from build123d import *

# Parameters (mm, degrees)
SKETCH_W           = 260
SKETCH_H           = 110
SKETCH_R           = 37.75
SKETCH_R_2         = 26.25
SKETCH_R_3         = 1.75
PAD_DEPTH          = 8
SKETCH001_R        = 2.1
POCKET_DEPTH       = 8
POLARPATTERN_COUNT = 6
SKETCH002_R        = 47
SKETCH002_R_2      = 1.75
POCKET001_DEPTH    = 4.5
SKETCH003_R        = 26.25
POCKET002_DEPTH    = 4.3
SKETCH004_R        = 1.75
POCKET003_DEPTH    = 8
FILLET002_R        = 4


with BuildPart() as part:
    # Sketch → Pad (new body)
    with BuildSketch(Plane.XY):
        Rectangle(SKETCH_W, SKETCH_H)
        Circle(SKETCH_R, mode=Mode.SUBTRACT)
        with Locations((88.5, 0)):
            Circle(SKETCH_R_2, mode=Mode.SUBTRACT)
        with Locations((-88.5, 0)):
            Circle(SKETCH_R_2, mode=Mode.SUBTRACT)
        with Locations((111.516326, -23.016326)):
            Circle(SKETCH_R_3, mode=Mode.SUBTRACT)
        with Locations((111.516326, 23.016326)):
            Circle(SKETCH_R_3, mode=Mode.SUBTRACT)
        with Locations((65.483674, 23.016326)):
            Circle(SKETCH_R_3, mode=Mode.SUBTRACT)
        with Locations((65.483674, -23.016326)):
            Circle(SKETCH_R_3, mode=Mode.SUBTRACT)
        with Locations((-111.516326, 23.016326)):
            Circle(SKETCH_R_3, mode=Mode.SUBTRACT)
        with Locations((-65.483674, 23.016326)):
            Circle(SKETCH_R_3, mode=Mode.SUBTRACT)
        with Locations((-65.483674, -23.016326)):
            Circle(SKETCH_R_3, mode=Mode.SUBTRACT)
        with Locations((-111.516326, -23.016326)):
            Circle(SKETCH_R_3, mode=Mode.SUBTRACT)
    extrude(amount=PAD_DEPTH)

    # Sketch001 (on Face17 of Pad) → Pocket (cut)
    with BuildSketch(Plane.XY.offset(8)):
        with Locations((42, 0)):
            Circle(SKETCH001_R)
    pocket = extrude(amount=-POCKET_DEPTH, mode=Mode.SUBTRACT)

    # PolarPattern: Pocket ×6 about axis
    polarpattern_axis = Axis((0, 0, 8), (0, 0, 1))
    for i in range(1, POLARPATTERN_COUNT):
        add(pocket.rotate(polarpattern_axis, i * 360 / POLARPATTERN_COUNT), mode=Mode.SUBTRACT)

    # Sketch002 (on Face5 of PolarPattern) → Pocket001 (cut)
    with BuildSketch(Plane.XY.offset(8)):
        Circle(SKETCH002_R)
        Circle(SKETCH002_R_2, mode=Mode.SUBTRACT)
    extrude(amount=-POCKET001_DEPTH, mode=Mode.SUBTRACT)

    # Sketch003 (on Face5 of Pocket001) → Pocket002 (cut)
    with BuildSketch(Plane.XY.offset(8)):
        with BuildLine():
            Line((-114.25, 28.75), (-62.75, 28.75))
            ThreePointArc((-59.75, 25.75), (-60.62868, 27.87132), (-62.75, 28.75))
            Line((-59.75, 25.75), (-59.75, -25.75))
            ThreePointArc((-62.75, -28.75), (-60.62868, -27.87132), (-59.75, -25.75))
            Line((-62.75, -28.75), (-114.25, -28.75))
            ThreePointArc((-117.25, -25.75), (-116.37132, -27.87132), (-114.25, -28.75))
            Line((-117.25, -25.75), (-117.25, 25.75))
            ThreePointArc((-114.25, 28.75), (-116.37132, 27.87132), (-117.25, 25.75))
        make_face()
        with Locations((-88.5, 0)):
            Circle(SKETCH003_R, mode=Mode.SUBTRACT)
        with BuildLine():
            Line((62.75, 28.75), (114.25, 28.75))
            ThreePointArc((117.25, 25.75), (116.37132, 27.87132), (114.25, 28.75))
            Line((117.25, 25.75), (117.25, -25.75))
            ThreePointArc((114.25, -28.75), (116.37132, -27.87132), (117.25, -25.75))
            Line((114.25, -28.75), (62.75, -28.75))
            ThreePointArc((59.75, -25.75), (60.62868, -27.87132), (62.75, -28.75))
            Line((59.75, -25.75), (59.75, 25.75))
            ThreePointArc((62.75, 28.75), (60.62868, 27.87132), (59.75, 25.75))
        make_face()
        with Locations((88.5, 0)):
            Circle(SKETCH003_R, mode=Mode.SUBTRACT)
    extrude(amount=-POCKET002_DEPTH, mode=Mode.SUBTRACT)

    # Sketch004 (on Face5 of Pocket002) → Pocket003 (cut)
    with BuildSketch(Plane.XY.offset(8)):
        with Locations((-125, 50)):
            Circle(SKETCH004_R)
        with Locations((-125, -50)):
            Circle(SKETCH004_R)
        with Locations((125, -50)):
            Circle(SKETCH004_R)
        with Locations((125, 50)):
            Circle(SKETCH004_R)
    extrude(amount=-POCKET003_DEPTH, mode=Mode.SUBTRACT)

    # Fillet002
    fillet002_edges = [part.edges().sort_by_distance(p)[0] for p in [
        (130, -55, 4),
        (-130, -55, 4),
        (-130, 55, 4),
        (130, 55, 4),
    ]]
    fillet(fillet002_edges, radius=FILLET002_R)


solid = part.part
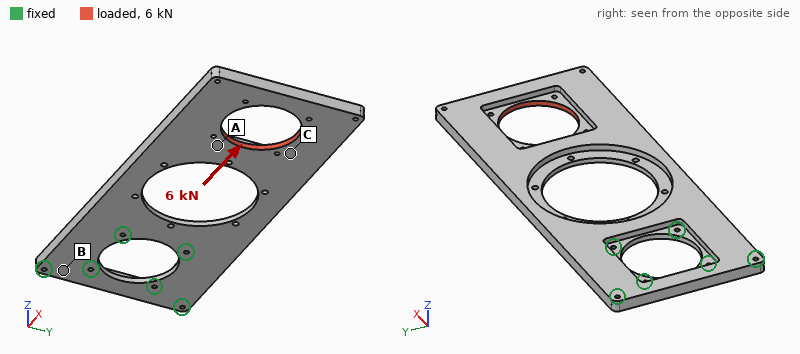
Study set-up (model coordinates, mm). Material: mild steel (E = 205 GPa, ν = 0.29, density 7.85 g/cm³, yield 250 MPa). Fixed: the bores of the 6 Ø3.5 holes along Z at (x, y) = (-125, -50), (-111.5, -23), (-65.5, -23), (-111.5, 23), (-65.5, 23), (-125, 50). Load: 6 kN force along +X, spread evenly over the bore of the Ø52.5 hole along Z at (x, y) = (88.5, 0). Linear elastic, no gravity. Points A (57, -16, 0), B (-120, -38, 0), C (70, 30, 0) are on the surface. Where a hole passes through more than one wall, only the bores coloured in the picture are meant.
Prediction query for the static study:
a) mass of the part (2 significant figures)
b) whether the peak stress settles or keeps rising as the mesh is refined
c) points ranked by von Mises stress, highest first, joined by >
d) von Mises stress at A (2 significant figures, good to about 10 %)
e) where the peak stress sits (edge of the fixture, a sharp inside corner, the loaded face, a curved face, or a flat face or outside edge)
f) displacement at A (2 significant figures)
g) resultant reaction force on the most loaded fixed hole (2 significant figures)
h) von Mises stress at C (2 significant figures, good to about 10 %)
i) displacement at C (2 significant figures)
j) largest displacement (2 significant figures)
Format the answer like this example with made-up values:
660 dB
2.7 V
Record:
1.1 kg
keeps rising
C > A > B
15 MPa
edge of the fixture
0.23 mm
1.5 kN
21 MPa
0.28 mm
0.53 mm
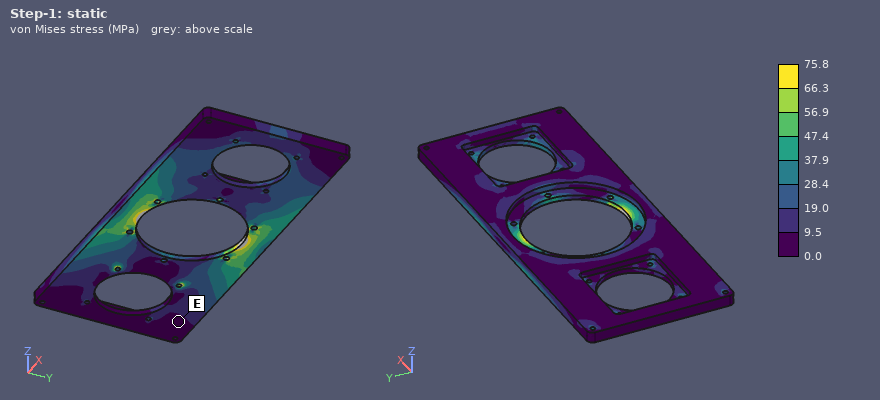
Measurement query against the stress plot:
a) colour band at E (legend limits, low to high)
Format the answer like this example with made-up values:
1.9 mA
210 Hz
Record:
0.0 to 9.5 MPa
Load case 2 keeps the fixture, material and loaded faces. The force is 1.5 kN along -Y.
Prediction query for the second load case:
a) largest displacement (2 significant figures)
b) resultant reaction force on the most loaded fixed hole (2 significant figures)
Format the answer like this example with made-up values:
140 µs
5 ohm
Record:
91 µm
1.5 kN
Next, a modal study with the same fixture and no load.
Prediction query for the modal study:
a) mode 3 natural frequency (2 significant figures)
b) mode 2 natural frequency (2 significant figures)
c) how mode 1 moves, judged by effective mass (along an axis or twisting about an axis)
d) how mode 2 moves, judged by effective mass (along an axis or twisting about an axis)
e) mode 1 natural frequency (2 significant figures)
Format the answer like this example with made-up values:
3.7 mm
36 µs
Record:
830 Hz
410 Hz
along Z
twisting about X
120 Hz
